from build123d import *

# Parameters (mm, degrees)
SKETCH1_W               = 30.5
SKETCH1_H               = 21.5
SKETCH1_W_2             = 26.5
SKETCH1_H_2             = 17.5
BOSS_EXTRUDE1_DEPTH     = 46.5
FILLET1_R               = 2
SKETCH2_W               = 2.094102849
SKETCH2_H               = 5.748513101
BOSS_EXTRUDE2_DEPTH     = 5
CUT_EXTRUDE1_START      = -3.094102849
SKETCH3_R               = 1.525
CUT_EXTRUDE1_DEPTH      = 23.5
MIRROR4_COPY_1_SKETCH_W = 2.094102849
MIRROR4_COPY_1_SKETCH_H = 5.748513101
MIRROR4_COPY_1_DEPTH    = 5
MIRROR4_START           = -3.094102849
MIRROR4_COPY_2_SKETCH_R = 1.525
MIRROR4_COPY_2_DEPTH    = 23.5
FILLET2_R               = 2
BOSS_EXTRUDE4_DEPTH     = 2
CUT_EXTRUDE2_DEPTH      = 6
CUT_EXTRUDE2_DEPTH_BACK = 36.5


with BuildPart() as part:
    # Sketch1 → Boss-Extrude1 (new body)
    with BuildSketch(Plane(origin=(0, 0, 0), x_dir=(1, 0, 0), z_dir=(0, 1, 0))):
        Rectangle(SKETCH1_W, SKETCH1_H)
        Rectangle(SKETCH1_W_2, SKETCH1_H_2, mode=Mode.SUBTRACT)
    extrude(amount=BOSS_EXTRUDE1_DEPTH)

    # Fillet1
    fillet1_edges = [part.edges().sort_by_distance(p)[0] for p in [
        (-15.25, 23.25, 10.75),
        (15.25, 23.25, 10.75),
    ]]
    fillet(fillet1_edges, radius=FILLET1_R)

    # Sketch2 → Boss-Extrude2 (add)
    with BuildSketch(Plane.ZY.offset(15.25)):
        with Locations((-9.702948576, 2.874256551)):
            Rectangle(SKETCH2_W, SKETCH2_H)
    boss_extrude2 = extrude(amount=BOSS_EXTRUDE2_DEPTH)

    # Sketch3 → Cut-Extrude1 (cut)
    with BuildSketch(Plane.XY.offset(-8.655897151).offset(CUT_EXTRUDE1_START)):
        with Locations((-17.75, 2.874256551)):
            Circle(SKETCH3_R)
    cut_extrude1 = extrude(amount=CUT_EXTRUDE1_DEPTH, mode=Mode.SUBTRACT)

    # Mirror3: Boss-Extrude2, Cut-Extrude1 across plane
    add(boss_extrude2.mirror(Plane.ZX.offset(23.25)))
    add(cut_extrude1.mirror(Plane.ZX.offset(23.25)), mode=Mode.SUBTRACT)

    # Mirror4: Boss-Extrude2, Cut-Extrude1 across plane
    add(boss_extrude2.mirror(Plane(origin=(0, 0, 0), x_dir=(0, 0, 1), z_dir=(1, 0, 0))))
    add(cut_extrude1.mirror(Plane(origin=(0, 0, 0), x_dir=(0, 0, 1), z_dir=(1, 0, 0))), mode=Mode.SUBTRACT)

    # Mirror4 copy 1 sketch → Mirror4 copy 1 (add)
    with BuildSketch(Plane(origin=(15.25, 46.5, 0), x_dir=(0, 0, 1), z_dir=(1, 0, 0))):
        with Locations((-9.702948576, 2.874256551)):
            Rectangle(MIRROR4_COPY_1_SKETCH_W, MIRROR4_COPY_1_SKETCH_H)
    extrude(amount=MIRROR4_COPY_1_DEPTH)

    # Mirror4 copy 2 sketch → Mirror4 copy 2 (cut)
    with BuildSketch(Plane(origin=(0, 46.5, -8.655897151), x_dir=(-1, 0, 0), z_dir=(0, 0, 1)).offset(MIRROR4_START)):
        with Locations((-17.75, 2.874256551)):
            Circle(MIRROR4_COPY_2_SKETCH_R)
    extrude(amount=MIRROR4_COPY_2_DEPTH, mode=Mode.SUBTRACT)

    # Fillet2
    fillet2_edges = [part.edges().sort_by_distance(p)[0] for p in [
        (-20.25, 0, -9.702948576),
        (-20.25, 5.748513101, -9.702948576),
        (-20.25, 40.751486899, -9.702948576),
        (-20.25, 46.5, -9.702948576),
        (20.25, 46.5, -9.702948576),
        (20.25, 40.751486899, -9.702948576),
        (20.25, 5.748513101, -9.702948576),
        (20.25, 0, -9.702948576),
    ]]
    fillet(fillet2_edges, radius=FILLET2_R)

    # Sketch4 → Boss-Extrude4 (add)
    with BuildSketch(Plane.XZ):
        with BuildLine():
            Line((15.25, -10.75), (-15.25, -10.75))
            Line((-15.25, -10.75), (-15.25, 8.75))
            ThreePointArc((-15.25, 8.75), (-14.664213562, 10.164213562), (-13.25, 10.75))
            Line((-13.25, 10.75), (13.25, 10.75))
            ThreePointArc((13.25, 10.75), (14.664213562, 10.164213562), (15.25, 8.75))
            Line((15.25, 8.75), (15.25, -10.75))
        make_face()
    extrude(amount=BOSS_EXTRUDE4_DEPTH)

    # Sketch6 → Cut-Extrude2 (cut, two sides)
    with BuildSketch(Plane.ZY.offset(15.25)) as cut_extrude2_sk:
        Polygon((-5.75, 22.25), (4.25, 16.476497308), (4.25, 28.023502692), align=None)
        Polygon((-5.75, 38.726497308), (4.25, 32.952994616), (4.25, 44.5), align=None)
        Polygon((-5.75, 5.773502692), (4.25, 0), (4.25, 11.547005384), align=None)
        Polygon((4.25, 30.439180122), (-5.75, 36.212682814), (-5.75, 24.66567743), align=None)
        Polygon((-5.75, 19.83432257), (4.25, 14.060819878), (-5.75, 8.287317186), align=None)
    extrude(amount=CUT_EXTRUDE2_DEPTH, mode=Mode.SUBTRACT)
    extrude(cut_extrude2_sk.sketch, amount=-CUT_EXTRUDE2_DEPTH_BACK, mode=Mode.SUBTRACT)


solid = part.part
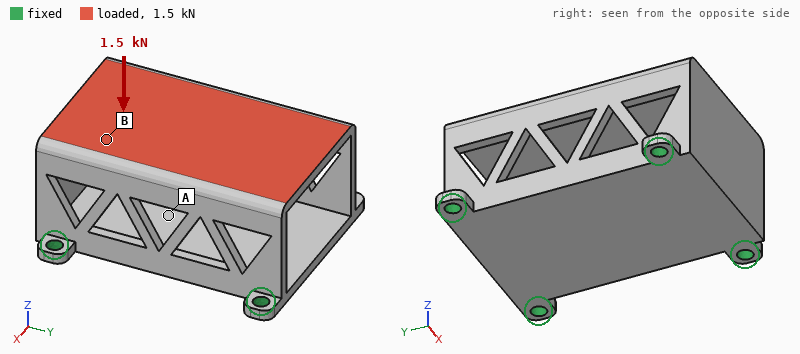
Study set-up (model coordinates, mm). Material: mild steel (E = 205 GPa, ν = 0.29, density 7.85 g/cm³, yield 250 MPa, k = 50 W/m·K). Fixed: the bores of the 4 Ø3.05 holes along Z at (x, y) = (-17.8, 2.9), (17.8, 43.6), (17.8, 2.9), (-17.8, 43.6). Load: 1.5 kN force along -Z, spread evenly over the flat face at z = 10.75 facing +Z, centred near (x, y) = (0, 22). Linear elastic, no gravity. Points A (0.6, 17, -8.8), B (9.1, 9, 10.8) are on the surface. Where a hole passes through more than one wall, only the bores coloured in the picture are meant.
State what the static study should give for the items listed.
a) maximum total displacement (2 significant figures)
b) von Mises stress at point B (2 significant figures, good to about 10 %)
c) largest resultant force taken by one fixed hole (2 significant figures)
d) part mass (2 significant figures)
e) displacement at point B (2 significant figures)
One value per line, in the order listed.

43 µm
45 MPa
400 N
72 g
14 µm
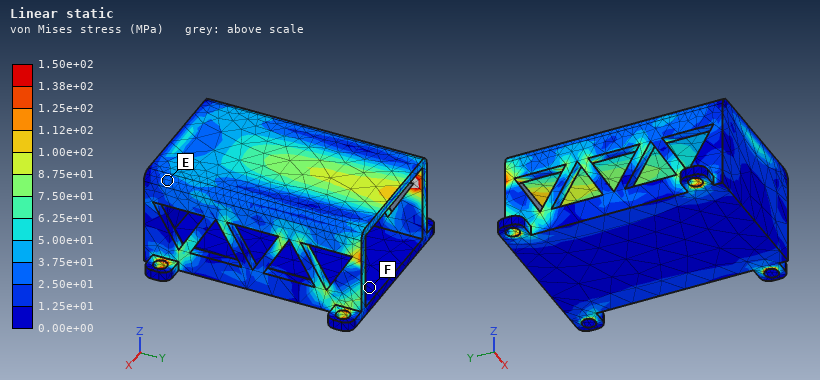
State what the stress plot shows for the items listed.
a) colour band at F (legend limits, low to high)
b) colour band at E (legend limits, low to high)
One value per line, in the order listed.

0.00e+00 to 1.25e+01 MPa
2.50e+01 to 3.75e+01 MPa
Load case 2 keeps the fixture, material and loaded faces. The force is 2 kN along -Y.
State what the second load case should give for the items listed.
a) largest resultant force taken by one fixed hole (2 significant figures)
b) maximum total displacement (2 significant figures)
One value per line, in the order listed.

710 N
23 µm
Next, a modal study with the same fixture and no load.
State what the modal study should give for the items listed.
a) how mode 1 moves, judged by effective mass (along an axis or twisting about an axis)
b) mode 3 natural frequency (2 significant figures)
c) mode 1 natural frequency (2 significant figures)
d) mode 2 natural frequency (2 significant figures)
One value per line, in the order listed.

along X
7600 Hz
4600 Hz
7500 Hz
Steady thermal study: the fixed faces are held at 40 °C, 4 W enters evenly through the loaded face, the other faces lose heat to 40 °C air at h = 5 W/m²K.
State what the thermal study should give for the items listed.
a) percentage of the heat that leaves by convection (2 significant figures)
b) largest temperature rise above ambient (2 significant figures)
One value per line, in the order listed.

11 %
21 K
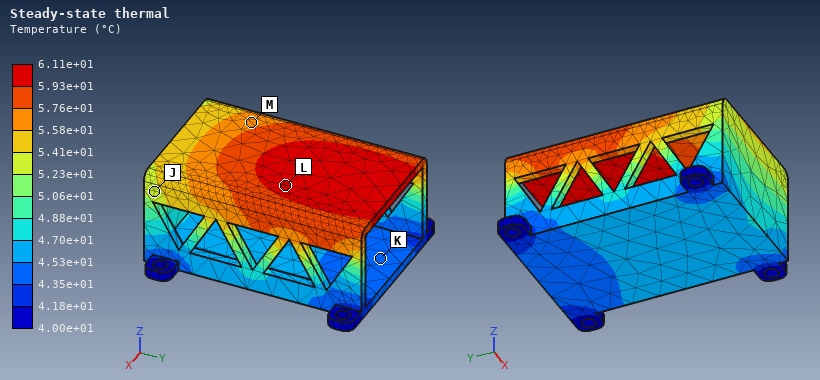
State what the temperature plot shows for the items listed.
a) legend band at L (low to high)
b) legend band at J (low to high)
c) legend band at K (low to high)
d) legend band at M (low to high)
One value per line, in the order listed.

5.93e+01 to 6.11e+01 °C
5.23e+01 to 5.41e+01 °C
4.35e+01 to 4.53e+01 °C
5.58e+01 to 5.76e+01 °C
